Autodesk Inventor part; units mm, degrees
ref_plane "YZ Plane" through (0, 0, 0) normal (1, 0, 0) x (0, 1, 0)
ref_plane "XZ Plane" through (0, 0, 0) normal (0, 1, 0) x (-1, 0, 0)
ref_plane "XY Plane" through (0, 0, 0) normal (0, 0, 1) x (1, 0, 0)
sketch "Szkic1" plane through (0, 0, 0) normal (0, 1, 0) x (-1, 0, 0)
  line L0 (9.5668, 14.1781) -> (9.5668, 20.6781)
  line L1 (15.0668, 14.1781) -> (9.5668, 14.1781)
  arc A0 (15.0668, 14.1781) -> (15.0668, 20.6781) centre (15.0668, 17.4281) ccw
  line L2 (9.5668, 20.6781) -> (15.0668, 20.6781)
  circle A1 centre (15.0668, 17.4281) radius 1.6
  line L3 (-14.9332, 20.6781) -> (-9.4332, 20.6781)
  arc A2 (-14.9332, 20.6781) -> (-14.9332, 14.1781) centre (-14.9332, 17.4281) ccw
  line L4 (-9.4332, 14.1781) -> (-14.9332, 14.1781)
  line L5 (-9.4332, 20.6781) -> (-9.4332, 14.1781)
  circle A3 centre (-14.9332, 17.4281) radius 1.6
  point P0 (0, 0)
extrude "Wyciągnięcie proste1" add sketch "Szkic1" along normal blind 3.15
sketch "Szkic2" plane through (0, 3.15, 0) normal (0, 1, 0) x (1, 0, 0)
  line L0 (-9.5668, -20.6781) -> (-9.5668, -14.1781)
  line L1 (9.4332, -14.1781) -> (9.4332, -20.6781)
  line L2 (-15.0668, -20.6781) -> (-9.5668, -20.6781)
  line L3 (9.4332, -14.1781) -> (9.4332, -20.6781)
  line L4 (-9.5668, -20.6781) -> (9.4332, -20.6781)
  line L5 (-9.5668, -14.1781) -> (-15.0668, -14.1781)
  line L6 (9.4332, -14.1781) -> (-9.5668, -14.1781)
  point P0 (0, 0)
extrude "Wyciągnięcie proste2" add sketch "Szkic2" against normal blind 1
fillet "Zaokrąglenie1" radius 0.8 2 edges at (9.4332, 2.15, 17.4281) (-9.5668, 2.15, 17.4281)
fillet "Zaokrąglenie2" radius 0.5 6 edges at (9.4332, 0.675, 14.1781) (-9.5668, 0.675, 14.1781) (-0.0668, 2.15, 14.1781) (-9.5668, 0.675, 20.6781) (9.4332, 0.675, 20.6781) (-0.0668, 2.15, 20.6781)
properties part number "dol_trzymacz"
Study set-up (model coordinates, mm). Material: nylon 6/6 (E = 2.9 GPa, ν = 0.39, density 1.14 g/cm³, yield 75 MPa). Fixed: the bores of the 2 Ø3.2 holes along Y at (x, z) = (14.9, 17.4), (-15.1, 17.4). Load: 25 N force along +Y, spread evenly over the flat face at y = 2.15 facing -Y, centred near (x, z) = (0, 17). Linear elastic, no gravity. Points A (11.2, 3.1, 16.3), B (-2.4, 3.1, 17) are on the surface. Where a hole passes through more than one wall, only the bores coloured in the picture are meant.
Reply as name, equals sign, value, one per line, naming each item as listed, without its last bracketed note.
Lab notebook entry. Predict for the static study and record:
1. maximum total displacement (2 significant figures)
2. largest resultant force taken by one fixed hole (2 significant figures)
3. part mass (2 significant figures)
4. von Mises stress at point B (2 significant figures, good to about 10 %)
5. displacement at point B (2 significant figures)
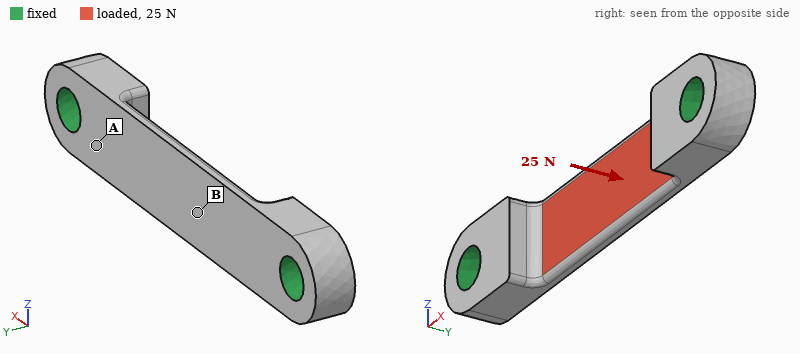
maximum total displacement = 0.37 mm
largest resultant force taken by one fixed hole = 17 N
part mass = 0.46 g
von Mises stress at point B = 18 MPa
displacement at point B = 0.32 mm
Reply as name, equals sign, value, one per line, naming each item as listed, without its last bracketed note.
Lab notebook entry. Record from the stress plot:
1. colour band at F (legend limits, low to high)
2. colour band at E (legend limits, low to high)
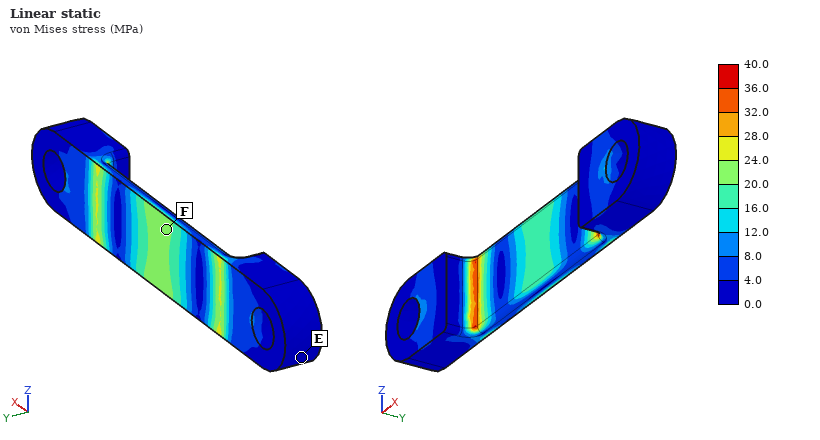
colour band at F = 20.0 to 24.0 MPa
colour band at E = 0.0 to 4.0 MPa
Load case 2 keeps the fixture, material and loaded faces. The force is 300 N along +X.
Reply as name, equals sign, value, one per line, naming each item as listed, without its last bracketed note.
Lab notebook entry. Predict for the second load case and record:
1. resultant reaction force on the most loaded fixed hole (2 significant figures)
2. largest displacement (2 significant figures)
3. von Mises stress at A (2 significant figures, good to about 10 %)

resultant reaction force on the most loaded fixed hole = 150 N
largest displacement = 96 µm
von Mises stress at A = 25 MPa
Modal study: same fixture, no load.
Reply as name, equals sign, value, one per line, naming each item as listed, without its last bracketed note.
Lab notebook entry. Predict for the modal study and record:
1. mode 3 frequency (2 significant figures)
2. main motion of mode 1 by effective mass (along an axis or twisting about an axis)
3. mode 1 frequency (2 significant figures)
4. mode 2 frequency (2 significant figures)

mode 3 frequency = 11 kHz
main motion of mode 1 by effective mass = along Y
mode 1 frequency = 4200 Hz
mode 2 frequency = 8500 Hz
